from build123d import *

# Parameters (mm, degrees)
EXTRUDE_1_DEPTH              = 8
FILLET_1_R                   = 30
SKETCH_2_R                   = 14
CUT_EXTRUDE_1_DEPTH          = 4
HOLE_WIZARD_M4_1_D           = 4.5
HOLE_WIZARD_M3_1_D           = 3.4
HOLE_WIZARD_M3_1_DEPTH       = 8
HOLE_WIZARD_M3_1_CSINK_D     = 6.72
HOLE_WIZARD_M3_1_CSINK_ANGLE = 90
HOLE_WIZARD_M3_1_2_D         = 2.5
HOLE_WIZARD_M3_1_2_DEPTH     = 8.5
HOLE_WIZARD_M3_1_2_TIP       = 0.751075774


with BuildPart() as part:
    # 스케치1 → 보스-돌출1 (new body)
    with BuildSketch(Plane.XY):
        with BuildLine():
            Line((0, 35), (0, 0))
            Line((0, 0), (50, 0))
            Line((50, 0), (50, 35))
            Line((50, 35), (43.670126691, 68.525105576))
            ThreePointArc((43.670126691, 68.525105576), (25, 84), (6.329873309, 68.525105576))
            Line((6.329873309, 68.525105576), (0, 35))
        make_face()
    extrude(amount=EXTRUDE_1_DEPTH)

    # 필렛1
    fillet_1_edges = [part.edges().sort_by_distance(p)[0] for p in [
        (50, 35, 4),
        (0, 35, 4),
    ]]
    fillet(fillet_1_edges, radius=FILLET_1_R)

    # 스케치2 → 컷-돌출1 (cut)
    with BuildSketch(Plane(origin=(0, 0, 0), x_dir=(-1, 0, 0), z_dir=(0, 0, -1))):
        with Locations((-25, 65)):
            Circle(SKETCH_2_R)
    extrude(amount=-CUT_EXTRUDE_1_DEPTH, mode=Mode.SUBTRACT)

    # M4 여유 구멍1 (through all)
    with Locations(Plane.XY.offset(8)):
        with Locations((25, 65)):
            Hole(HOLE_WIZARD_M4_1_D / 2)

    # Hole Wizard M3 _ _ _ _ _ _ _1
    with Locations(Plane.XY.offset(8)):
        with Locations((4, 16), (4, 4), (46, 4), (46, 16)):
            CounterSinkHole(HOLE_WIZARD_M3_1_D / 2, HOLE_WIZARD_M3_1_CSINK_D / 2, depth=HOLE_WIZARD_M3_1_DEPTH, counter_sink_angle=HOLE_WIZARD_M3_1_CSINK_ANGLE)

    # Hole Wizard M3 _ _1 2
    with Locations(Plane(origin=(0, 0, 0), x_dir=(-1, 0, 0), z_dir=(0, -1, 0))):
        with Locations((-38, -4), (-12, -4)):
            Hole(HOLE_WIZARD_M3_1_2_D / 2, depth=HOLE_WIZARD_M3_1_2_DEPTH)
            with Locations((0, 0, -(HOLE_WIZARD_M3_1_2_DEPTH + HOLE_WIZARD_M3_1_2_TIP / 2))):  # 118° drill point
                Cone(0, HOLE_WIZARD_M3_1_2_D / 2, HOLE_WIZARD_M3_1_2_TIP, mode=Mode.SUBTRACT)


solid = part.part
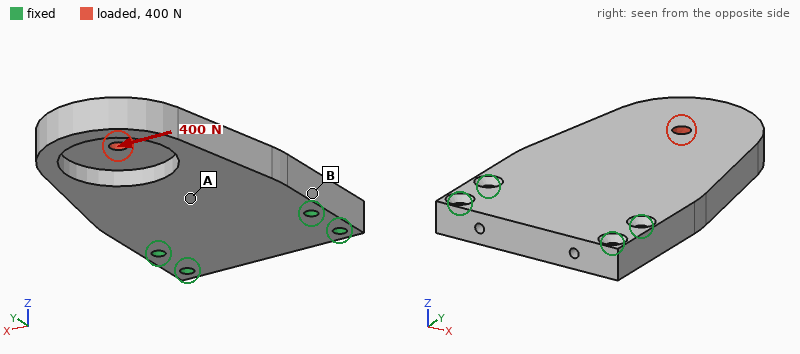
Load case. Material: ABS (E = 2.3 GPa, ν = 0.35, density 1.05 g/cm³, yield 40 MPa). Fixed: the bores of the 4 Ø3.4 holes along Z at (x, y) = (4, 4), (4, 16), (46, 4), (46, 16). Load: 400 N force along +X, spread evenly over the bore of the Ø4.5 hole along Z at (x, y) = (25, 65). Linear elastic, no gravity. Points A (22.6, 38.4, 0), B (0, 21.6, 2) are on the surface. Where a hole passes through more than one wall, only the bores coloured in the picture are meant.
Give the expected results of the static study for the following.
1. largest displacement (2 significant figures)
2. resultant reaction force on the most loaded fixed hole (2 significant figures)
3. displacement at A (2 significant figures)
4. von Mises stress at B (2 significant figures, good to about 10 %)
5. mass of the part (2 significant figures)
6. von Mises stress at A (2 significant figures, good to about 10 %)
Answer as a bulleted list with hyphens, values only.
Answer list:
- 0.24 mm
- 440 N
- 0.051 mm
- 5.7 MPa
- 28 g
- 1.8 MPa
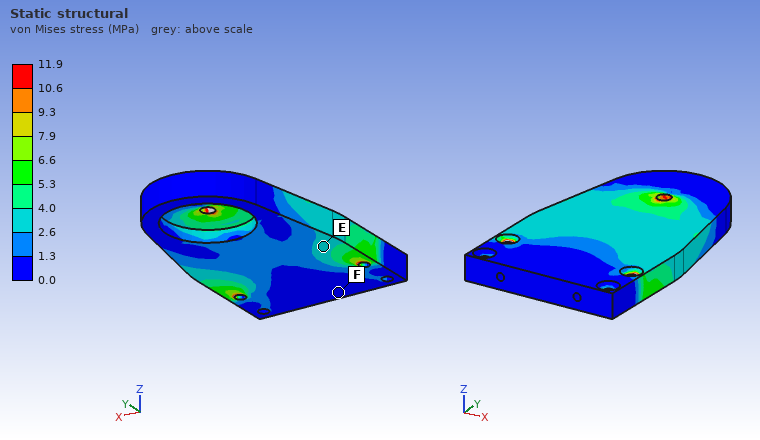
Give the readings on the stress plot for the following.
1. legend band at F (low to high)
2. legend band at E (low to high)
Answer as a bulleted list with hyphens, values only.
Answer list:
- 0.0 to 1.3 MPa
- 2.6 to 4.0 MPa
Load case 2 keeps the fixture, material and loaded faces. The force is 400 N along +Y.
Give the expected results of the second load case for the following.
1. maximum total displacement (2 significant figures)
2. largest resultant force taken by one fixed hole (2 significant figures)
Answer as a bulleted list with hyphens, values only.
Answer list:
- 0.42 mm
- 150 N
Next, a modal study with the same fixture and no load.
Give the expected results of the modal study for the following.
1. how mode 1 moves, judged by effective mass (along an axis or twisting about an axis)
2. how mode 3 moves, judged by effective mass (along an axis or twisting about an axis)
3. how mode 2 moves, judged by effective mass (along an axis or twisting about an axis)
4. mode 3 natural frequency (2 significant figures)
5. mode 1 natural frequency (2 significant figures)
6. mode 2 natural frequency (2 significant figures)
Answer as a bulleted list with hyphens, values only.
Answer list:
- along Z
- along Z
- twisting about Y
- 2100 Hz
- 500 Hz
- 1600 Hz
